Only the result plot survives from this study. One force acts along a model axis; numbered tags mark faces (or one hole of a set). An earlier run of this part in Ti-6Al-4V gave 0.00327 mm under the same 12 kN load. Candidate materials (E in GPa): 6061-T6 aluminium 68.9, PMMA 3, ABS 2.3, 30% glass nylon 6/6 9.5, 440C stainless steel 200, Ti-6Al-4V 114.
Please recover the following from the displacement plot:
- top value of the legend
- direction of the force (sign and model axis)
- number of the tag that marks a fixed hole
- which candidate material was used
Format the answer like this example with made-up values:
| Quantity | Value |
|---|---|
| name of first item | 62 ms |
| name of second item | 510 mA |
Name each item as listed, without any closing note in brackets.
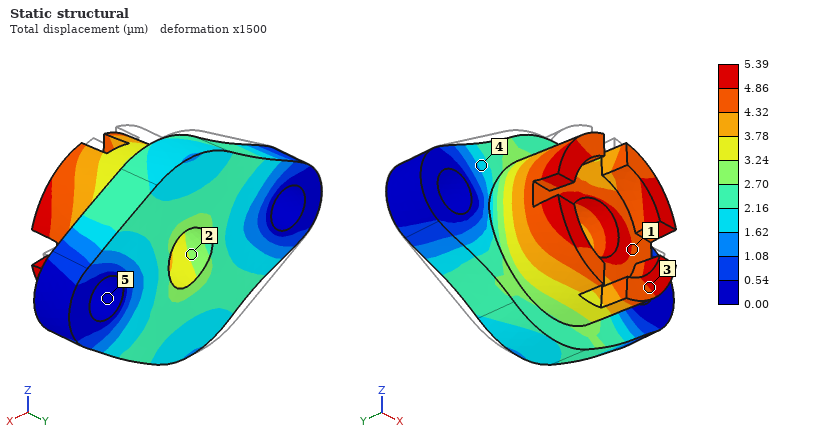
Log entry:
| Quantity | Value |
|---|---|
| top value of the legend | 5.39 µm |
| direction of the force | +X |
| number of the tag that marks a fixed hole | 5 |
| which candidate material was used | 6061-T6 aluminium |
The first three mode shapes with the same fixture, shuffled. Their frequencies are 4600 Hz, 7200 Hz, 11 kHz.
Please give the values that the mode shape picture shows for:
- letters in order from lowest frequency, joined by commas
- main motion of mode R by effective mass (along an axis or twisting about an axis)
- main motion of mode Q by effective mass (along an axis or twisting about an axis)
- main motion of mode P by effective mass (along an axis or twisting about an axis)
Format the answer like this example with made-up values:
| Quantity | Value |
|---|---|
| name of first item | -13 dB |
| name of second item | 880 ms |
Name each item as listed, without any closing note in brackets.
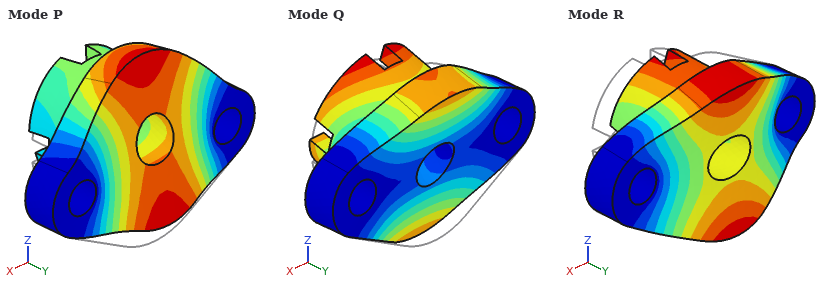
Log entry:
| Quantity | Value |
|---|---|
| letters in order from lowest frequency, joined by commas | Q, R, P |
| main motion of mode R by effective mass | along Y |
| main motion of mode Q by effective mass | along Z |
| main motion of mode P by effective mass | along Z |
